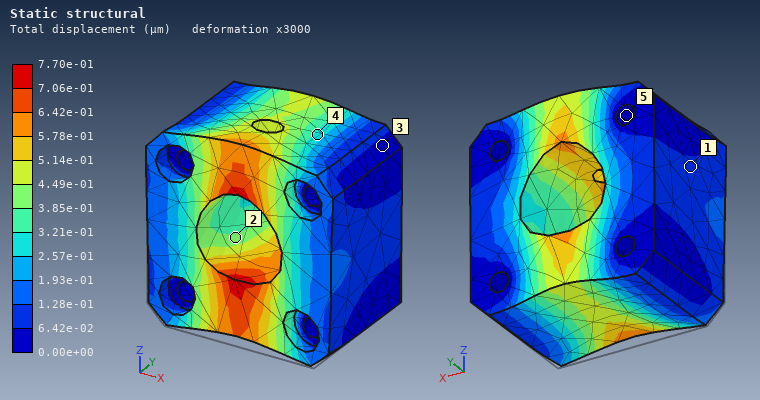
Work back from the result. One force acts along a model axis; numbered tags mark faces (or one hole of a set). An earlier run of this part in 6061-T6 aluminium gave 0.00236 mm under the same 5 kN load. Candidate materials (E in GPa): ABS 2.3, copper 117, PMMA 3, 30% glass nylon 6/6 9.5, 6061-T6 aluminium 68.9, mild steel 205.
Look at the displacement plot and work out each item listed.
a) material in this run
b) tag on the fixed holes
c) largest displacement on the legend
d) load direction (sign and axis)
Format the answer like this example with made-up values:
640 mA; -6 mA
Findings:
mild steel; 5; 7.70e-01 µm; +Z
